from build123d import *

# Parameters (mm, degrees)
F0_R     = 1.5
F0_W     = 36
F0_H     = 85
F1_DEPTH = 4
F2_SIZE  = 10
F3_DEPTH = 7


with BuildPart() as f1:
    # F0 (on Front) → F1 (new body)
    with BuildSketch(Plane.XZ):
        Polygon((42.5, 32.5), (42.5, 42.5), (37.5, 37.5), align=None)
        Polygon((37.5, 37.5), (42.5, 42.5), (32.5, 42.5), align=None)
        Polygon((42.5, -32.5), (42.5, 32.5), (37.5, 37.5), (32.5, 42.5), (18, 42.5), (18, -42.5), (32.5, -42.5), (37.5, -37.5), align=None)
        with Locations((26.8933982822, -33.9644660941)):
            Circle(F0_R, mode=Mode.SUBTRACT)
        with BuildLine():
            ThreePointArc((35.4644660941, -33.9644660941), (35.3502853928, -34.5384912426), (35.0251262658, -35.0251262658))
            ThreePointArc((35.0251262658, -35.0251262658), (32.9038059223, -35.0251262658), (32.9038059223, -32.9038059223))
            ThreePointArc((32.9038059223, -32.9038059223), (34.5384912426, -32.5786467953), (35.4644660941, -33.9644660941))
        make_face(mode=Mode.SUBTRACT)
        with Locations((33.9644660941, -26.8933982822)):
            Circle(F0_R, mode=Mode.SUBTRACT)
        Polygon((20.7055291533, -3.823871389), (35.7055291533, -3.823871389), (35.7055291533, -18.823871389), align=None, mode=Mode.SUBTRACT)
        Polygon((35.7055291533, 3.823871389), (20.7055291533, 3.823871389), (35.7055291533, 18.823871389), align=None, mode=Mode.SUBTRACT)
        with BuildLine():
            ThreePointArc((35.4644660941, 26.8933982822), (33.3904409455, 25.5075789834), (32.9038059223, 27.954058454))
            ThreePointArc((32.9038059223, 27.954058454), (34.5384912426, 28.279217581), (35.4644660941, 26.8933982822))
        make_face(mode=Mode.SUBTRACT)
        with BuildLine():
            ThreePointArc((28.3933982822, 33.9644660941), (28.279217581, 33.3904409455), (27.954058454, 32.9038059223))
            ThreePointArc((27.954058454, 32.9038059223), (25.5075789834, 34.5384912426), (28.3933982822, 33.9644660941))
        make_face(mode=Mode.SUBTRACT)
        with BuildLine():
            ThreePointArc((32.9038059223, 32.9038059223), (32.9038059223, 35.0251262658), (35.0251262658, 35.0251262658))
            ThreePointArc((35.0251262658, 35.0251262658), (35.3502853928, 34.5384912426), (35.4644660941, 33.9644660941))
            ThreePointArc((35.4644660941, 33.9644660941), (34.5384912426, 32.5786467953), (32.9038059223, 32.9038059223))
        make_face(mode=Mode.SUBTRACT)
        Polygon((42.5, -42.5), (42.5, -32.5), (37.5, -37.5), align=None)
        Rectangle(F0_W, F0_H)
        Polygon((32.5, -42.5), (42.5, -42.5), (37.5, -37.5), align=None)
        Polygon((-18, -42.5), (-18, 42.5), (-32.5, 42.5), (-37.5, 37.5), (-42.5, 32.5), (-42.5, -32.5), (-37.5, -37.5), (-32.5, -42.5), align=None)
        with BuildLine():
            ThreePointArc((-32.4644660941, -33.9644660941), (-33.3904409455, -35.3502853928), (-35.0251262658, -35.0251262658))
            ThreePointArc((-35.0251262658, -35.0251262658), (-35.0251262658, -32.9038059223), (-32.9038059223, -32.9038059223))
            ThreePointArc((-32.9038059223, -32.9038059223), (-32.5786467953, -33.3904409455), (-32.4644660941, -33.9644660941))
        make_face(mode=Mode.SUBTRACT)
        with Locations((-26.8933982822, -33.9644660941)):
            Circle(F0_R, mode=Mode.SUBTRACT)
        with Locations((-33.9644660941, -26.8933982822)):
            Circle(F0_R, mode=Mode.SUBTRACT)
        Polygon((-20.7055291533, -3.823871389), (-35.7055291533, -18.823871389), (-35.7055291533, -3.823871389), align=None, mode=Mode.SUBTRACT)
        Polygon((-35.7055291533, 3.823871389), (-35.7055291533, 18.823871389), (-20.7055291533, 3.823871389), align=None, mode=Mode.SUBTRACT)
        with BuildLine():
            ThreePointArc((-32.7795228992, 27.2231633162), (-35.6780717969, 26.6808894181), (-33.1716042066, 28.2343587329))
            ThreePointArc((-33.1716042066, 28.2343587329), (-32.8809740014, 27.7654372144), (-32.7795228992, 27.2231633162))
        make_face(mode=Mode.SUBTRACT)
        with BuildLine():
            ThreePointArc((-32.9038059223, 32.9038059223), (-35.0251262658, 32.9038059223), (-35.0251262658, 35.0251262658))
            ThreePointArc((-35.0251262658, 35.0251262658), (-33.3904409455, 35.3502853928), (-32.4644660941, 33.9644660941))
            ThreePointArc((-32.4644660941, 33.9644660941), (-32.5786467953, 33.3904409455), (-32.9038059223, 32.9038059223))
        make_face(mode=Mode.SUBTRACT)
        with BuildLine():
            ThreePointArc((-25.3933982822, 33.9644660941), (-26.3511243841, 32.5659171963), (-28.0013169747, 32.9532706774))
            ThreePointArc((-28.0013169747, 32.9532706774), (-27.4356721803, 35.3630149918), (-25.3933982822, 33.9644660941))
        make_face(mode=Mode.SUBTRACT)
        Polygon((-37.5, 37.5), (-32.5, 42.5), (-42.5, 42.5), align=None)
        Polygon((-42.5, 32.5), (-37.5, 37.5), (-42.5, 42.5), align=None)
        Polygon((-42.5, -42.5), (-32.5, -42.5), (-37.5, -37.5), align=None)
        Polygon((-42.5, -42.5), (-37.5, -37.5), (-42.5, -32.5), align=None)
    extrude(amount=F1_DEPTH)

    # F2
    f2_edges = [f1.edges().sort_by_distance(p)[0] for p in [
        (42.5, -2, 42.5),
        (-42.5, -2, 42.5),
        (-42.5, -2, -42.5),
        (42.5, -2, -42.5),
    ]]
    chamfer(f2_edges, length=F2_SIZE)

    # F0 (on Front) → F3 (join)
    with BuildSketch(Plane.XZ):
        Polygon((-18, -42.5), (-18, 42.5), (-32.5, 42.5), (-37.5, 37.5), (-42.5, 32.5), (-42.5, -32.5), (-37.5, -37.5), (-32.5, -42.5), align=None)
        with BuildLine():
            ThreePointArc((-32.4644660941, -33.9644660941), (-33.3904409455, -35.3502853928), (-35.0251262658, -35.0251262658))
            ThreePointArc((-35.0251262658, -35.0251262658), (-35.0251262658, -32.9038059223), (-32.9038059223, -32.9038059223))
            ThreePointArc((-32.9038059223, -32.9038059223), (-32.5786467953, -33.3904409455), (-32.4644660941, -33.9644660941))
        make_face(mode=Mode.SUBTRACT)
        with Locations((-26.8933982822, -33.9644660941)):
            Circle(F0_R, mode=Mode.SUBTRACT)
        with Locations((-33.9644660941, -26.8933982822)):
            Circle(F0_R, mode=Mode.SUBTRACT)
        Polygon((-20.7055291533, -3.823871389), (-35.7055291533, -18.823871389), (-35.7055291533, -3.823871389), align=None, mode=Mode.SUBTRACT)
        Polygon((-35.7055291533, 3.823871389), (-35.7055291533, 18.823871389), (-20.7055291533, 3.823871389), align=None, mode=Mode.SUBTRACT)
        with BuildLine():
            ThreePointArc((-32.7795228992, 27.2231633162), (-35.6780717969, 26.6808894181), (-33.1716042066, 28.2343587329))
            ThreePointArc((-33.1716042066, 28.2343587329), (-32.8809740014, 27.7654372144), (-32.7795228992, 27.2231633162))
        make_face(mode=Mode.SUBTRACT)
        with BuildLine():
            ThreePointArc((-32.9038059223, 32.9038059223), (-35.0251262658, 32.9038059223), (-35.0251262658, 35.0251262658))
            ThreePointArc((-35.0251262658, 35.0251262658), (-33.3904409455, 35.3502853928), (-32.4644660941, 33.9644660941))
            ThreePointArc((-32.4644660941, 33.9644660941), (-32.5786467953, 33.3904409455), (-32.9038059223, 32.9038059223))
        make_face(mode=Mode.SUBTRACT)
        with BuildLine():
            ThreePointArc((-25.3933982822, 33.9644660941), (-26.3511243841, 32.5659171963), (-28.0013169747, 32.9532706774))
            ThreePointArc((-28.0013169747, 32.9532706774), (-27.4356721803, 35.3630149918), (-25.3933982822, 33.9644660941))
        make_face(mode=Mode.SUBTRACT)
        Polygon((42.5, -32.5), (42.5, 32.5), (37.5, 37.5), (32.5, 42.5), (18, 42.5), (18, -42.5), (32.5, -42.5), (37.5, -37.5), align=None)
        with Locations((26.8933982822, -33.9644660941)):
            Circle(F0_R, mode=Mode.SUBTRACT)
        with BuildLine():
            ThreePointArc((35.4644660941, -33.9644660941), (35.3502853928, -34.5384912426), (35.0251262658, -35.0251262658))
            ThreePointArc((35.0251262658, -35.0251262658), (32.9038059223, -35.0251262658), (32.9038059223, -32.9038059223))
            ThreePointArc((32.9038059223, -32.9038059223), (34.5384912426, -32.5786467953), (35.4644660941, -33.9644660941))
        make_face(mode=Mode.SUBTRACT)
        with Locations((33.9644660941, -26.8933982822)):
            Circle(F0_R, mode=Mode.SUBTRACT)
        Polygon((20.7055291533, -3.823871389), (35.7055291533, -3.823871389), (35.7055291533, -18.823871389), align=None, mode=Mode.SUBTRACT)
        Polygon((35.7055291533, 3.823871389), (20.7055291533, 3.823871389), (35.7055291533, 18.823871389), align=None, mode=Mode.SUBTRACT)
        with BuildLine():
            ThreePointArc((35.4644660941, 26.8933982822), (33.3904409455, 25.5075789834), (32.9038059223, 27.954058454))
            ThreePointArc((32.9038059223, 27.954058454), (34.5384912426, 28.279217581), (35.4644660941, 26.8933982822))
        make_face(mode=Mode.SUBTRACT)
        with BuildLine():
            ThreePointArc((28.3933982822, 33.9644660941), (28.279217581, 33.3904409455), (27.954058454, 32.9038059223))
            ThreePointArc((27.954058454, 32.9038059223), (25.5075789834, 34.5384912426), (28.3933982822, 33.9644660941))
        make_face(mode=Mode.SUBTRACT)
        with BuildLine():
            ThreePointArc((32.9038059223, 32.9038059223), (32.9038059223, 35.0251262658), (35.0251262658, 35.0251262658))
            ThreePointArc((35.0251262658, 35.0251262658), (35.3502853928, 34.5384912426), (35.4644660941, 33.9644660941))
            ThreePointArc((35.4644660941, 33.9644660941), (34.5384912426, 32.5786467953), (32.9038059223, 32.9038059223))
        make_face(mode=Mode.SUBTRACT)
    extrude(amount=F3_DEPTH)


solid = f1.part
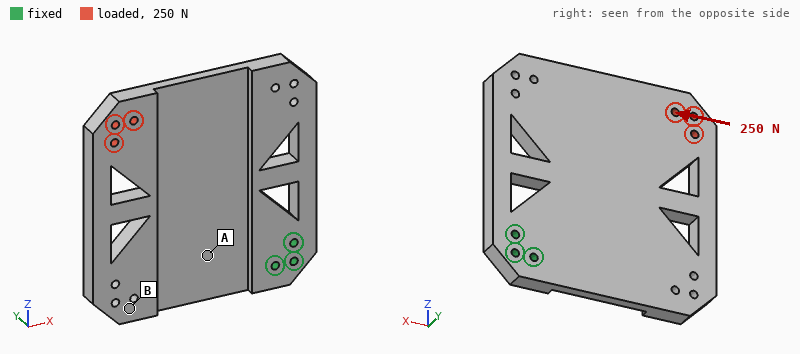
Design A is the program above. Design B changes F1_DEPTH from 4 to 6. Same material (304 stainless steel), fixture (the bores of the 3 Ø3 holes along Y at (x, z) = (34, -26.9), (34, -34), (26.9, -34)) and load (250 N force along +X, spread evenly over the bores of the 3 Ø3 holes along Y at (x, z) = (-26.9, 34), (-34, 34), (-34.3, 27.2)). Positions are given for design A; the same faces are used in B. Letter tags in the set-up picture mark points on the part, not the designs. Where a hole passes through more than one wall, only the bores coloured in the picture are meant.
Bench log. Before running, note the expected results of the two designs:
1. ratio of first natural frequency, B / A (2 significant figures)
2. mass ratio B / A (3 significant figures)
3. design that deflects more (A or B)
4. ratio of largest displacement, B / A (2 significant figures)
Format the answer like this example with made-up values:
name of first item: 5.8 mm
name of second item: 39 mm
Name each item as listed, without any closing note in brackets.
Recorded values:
ratio of first natural frequency, B / A: 1.2
mass ratio B / A: 1.17
design that deflects more: A
ratio of largest displacement, B / A: 0.86
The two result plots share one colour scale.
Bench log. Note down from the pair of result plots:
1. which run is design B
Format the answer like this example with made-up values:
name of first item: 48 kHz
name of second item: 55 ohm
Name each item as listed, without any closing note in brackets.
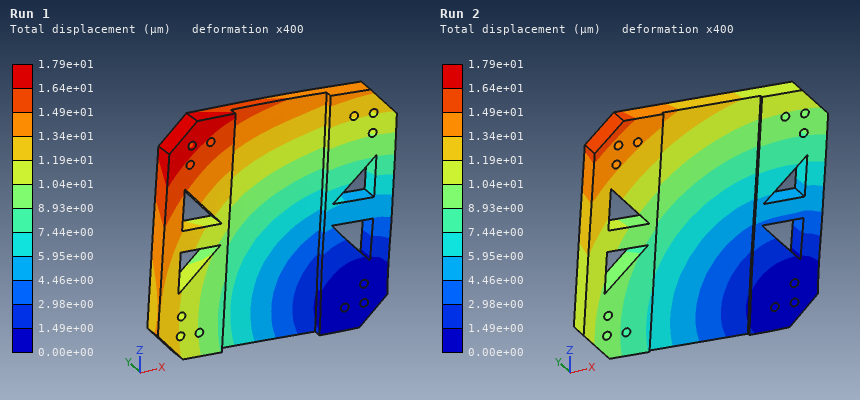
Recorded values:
which run is design B: Run 2
